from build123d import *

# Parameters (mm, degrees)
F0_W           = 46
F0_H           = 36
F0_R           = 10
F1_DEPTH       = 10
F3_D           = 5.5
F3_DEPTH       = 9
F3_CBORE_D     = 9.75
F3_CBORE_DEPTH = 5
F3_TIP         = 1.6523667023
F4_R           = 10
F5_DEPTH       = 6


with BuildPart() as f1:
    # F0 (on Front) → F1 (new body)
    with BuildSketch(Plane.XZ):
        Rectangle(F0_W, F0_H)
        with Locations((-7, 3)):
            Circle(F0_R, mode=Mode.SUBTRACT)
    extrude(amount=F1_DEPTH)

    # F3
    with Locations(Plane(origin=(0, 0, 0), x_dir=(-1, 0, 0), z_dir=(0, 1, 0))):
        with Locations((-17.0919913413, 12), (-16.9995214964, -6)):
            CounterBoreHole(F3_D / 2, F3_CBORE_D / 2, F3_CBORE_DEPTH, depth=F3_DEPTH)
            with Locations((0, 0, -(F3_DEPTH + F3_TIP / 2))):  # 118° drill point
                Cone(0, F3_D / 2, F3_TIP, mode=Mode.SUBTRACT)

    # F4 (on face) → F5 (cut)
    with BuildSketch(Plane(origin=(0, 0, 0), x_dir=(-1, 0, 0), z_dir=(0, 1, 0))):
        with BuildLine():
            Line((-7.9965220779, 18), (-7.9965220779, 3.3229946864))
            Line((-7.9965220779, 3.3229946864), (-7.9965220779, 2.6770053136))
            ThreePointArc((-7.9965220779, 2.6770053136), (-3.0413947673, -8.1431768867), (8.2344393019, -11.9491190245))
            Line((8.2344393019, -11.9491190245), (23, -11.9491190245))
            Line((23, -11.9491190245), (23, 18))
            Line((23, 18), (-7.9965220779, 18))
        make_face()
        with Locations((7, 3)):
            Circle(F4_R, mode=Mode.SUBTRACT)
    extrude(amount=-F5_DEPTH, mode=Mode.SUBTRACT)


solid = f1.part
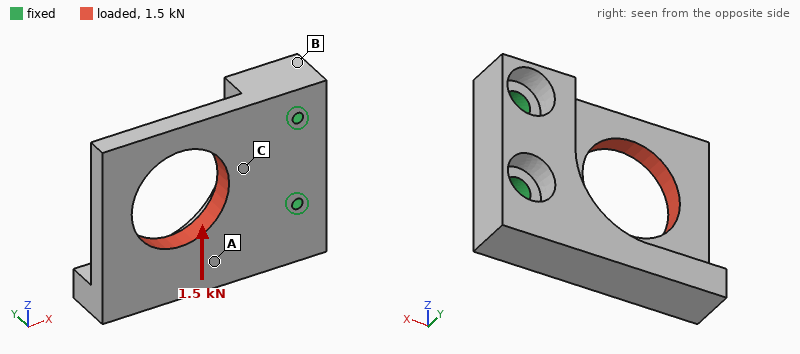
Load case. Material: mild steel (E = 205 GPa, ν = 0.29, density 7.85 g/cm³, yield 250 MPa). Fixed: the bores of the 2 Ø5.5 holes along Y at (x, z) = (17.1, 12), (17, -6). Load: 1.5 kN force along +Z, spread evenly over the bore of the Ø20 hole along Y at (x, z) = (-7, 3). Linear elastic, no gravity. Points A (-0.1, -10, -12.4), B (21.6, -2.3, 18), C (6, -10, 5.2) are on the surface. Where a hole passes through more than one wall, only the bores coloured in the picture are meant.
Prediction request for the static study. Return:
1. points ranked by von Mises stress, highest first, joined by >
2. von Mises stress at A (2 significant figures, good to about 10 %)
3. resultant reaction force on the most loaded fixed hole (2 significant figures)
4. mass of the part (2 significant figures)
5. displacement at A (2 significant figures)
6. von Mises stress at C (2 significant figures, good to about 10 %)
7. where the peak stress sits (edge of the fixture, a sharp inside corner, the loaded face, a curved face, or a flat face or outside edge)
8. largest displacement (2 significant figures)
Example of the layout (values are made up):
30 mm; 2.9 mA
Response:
C > A > B; 23 MPa; 1.7 kN; 71 g; 5.9 µm; 45 MPa; edge of the fixture; 21 µm
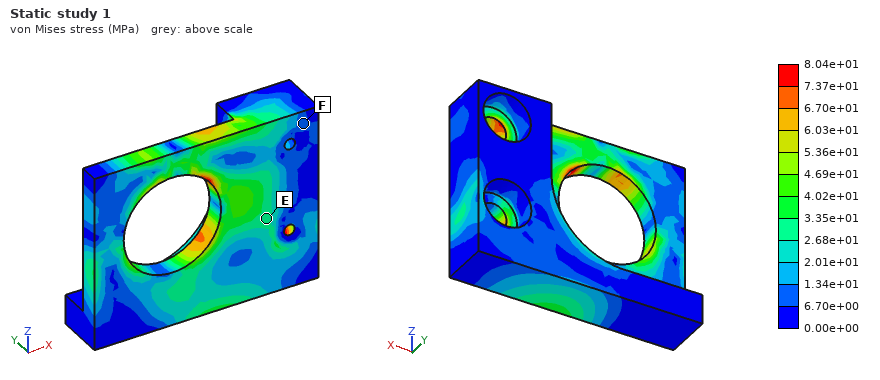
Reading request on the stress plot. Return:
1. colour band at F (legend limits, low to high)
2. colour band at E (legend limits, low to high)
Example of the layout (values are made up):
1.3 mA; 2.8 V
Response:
6.70e+00 to 1.34e+01 MPa; 2.68e+01 to 3.35e+01 MPa
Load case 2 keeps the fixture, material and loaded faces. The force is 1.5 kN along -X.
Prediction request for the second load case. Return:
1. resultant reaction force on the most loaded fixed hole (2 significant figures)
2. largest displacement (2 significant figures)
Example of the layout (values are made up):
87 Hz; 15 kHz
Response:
770 N; 6.5 µm
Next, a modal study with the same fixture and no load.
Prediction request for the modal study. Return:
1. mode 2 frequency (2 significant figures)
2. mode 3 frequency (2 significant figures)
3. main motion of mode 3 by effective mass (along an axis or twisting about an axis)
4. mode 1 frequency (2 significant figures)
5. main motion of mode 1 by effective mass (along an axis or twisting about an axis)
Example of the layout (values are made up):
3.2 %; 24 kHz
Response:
5800 Hz; 8500 Hz; along Z; 3500 Hz; along Y
